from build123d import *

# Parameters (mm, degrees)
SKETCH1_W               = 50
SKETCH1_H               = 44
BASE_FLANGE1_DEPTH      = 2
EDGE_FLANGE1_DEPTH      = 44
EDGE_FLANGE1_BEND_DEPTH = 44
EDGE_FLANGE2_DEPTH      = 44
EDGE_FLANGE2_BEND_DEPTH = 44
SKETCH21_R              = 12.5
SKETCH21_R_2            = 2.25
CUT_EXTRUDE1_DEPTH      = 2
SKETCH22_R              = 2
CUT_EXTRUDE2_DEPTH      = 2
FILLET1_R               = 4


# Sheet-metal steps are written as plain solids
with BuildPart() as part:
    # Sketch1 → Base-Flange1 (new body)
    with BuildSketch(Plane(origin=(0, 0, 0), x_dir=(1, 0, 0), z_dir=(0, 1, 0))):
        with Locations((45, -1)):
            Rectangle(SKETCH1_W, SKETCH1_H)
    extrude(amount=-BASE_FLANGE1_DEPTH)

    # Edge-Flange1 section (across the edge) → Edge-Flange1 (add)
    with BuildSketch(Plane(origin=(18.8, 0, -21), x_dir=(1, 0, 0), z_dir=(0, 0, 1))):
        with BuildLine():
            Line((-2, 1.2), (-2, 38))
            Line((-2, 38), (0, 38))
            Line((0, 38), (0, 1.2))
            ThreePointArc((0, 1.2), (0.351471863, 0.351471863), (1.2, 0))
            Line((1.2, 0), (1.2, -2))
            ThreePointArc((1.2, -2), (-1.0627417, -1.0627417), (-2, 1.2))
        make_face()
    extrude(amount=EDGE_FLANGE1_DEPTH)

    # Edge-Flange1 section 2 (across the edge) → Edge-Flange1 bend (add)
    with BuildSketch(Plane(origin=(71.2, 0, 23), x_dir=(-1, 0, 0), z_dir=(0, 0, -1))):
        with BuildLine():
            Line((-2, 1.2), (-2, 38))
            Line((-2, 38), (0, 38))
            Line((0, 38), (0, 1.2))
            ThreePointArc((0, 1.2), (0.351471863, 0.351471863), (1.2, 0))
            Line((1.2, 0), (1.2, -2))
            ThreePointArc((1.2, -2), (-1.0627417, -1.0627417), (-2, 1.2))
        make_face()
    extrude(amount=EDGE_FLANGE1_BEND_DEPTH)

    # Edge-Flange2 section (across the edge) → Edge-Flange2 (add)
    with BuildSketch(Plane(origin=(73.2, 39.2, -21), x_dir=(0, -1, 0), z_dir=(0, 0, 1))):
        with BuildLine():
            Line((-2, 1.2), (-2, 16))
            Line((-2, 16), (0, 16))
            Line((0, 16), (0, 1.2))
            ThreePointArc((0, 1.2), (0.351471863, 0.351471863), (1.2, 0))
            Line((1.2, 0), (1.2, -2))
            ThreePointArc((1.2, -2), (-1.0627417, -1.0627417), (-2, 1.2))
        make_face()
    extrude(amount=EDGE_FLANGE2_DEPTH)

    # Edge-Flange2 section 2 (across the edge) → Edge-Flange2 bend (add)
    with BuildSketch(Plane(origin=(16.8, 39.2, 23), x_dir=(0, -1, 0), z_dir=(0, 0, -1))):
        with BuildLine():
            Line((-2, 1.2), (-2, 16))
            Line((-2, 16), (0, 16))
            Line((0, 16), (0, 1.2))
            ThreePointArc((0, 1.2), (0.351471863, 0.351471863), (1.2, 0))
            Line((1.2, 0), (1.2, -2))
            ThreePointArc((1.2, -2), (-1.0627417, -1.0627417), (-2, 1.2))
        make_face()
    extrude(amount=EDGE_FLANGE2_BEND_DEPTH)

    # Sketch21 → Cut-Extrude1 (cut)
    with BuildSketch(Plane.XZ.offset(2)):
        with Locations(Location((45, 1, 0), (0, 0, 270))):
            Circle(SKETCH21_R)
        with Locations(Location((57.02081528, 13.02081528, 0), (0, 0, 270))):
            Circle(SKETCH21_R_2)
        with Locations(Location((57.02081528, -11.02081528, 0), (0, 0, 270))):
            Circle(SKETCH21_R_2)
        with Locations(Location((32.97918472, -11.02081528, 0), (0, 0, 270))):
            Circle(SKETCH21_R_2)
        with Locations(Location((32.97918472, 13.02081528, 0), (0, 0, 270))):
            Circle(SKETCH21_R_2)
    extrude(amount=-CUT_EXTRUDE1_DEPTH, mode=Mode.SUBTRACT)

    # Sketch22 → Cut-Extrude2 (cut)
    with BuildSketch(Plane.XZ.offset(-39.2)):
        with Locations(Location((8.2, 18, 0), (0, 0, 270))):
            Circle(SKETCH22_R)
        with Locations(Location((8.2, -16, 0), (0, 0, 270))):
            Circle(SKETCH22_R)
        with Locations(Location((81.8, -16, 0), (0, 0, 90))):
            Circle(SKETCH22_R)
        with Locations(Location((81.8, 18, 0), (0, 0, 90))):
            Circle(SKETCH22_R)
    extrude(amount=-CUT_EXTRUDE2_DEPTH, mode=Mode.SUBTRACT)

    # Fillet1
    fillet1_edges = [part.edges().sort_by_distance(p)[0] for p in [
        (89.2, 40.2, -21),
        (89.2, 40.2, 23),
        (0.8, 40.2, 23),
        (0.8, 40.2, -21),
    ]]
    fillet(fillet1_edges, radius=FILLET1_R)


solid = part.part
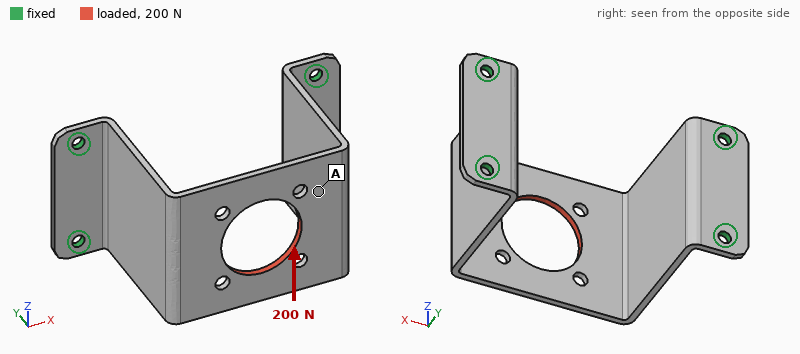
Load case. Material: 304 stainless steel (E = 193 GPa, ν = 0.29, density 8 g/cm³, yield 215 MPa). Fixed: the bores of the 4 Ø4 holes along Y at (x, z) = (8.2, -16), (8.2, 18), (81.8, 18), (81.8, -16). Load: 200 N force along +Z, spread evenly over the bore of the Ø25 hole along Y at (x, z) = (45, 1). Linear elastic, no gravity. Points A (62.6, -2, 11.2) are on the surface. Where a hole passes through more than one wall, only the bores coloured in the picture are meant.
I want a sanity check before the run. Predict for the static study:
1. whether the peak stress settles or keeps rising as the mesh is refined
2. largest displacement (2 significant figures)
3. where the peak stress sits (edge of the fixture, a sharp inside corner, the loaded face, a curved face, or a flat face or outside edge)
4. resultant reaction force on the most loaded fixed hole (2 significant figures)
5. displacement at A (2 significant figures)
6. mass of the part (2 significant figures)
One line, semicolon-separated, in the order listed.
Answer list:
keeps rising; 25 µm; edge of the fixture; 130 N; 23 µm; 110 g
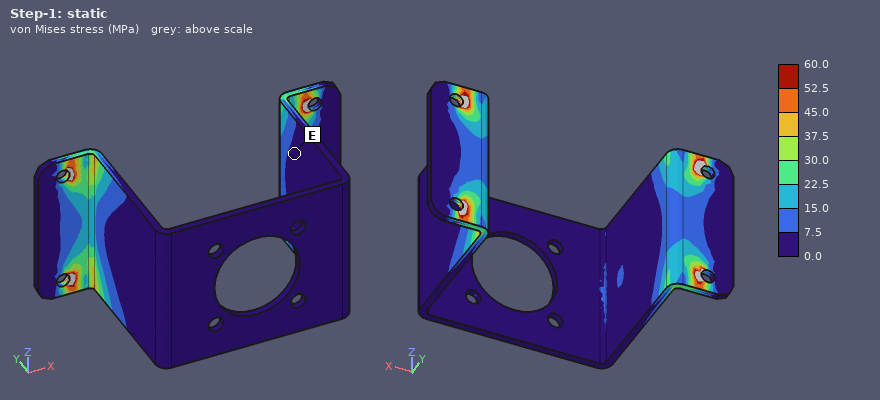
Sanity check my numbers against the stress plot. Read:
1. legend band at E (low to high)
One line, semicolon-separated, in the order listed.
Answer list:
0.0 to 7.5 MPa
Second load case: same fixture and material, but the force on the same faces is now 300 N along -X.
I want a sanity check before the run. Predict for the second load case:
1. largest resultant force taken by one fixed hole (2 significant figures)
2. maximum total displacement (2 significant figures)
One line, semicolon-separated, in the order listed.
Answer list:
97 N; 0.32 mm
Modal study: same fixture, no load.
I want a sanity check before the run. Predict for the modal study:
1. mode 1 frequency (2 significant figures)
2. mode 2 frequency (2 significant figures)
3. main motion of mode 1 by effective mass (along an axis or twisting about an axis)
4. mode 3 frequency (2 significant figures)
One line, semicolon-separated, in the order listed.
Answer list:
700 Hz; 2000 Hz; along X; 2000 Hz
